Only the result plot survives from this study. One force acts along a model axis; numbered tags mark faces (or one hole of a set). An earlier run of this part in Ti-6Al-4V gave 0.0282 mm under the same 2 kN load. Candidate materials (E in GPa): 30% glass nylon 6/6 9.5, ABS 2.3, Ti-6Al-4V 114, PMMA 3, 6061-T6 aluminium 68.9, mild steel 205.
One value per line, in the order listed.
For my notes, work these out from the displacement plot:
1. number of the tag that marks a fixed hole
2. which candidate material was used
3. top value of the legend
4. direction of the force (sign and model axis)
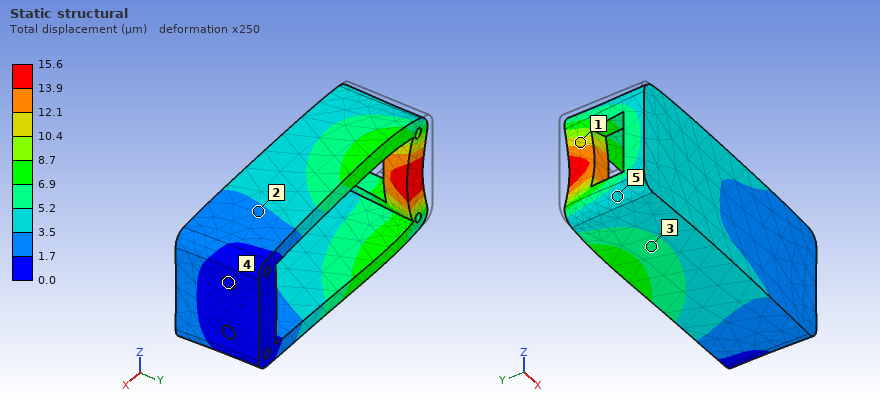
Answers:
4
mild steel
15.6 µm
+X
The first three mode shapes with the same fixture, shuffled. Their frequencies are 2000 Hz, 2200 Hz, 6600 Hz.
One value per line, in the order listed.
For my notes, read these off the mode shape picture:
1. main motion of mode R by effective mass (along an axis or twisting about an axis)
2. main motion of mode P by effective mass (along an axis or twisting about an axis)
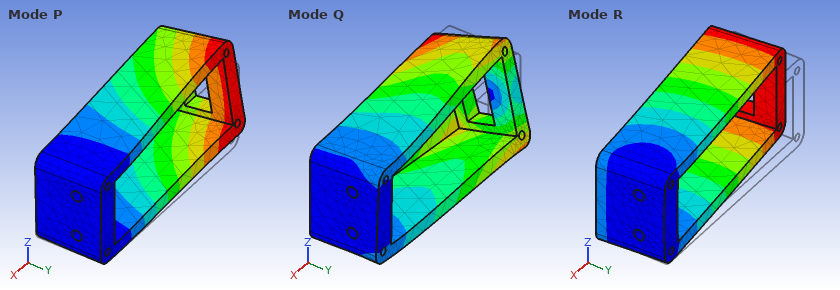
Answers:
along Y
along Z
